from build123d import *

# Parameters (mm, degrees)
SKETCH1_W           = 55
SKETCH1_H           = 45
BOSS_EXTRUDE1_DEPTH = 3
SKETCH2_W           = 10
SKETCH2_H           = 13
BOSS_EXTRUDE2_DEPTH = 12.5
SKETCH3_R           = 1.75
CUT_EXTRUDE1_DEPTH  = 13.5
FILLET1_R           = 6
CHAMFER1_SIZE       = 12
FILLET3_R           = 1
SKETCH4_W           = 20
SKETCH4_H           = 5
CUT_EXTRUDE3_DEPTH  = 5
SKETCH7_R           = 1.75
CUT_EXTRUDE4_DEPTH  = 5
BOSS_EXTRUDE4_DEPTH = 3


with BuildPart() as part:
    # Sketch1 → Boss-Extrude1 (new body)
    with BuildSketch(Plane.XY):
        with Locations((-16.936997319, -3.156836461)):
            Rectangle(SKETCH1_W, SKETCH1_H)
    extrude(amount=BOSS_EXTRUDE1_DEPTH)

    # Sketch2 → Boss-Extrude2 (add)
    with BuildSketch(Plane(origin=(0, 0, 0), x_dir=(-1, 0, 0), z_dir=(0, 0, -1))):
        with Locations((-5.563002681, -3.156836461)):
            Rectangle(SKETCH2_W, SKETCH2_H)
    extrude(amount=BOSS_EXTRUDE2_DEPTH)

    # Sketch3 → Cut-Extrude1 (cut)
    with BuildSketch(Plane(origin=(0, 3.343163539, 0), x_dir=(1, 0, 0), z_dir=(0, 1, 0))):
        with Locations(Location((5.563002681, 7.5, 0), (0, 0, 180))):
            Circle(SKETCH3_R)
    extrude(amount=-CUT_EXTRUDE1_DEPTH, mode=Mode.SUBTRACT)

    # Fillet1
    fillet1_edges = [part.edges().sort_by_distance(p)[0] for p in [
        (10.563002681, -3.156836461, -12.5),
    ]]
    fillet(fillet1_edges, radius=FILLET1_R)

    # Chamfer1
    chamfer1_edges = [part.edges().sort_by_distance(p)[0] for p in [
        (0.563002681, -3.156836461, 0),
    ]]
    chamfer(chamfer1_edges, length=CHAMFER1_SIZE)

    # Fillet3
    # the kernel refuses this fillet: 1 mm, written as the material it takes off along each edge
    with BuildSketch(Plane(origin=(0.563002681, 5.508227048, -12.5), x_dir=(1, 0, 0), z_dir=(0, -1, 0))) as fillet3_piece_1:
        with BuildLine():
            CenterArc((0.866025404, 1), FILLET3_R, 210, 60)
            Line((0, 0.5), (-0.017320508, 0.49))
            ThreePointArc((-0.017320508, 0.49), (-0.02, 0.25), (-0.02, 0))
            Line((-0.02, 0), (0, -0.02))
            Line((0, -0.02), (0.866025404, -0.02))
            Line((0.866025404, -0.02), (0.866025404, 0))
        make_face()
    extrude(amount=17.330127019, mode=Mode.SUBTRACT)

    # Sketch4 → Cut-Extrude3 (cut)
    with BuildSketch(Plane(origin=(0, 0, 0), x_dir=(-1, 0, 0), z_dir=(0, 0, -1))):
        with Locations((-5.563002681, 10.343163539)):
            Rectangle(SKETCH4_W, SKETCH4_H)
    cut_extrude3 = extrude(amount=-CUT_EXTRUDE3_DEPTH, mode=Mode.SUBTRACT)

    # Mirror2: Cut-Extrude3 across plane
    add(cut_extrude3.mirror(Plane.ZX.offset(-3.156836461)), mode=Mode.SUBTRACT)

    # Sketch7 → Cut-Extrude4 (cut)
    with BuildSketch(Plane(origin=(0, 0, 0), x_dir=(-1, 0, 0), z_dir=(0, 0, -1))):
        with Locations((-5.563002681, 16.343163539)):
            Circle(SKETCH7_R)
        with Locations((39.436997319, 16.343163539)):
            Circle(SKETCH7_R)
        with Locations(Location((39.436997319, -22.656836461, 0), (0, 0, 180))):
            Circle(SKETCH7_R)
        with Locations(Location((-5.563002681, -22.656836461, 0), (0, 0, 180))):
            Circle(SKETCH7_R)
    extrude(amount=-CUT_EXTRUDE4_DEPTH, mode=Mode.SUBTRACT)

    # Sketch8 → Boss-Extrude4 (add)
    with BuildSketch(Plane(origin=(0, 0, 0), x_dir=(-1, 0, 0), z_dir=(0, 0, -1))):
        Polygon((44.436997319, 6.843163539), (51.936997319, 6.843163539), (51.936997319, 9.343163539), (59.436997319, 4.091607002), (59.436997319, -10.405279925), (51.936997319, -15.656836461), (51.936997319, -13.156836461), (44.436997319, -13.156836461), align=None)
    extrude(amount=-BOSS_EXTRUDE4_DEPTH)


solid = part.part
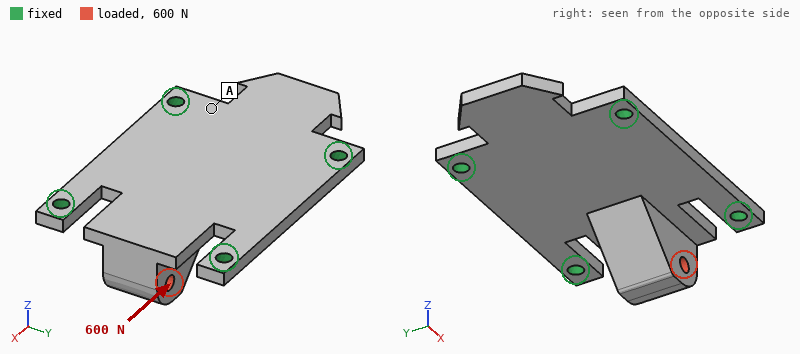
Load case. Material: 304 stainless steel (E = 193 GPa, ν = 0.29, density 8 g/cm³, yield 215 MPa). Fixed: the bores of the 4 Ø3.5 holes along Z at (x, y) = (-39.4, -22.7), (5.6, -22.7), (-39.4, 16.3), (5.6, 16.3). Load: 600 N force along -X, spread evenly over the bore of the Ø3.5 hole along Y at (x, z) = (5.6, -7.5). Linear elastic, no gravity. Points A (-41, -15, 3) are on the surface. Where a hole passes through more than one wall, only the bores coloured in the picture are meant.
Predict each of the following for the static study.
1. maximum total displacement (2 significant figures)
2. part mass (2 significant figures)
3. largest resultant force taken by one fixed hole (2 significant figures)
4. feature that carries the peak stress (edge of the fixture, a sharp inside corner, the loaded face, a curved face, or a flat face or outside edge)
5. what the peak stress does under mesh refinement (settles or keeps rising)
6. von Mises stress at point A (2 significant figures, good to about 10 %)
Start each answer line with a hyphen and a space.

- 67 µm
- 81 g
- 240 N
- a sharp inside corner
- keeps rising
- 13 MPa
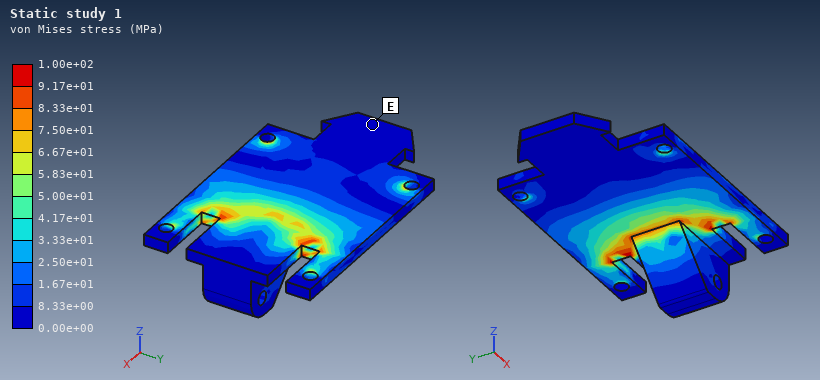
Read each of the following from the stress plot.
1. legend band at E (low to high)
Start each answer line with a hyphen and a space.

- 0.00e+00 to 8.33e+00 MPa
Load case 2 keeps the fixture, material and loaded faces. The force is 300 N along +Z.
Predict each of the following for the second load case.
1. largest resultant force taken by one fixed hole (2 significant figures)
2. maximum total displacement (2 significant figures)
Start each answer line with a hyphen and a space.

- 180 N
- 76 µm
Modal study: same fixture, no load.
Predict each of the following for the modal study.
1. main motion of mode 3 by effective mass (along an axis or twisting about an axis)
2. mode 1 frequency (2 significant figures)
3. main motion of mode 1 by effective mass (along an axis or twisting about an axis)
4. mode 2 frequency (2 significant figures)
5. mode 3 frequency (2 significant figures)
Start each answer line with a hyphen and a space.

- along Z
- 2300 Hz
- along Z
- 4100 Hz
- 5100 Hz
